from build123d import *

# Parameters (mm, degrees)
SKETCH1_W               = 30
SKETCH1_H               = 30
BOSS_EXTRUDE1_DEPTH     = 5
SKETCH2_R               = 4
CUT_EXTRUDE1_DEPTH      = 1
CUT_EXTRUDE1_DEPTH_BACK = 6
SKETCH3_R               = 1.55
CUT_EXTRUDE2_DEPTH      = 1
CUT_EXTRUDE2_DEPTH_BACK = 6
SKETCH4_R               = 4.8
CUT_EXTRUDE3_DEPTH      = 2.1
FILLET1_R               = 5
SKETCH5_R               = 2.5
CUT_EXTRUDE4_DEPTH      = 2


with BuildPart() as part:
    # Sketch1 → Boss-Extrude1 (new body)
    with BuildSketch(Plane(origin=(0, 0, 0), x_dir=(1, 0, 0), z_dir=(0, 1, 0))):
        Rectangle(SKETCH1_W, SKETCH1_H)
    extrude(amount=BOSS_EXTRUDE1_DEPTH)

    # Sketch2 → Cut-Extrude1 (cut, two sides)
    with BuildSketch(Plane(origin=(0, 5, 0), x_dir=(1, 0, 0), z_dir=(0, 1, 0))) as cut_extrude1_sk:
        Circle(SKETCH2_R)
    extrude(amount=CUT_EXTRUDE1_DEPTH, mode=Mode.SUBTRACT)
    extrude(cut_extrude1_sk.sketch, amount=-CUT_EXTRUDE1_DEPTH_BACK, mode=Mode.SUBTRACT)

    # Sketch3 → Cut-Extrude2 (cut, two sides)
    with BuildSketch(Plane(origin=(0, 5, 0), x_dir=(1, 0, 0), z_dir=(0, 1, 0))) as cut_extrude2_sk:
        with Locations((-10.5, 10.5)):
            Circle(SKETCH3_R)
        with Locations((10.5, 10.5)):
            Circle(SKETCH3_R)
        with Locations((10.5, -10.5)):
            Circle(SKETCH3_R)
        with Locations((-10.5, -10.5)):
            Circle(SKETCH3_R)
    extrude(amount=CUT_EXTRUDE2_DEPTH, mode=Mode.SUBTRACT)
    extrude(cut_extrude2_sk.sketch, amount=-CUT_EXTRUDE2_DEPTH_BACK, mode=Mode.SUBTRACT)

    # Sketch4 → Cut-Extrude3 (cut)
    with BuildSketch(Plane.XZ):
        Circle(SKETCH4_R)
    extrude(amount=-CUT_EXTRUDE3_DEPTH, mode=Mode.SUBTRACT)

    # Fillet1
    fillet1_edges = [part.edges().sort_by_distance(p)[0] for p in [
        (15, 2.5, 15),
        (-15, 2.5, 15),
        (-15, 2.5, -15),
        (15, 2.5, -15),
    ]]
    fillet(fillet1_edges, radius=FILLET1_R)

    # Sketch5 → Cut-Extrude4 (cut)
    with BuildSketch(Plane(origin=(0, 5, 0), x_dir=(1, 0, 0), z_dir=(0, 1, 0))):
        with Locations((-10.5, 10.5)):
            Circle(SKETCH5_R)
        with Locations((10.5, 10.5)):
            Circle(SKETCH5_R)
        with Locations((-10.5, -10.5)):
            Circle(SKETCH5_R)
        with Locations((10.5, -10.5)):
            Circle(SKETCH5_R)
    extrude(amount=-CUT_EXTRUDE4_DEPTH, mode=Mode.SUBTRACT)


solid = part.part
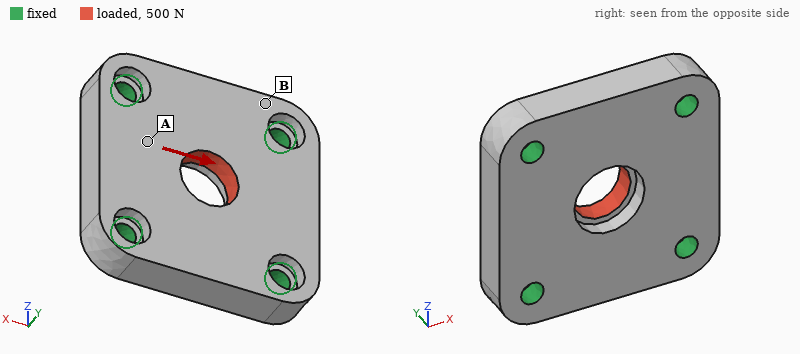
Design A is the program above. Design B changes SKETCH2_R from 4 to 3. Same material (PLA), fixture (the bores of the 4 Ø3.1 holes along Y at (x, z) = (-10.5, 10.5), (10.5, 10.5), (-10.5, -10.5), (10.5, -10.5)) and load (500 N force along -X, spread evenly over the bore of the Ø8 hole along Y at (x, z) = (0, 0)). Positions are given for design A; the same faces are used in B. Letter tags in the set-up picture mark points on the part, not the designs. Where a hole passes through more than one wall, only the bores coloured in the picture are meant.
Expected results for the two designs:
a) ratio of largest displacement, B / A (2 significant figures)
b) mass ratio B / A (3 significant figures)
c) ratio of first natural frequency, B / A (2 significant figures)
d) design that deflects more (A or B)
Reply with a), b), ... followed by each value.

a) 1.1
b) 1.02
c) 0.99
d) B
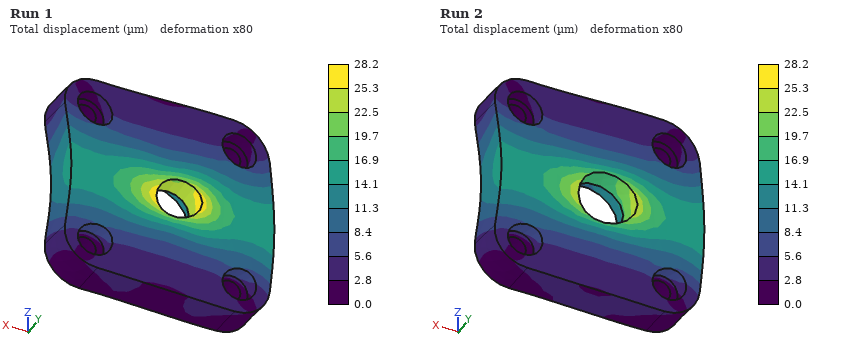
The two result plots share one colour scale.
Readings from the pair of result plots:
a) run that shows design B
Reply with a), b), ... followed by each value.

a) Run 1
